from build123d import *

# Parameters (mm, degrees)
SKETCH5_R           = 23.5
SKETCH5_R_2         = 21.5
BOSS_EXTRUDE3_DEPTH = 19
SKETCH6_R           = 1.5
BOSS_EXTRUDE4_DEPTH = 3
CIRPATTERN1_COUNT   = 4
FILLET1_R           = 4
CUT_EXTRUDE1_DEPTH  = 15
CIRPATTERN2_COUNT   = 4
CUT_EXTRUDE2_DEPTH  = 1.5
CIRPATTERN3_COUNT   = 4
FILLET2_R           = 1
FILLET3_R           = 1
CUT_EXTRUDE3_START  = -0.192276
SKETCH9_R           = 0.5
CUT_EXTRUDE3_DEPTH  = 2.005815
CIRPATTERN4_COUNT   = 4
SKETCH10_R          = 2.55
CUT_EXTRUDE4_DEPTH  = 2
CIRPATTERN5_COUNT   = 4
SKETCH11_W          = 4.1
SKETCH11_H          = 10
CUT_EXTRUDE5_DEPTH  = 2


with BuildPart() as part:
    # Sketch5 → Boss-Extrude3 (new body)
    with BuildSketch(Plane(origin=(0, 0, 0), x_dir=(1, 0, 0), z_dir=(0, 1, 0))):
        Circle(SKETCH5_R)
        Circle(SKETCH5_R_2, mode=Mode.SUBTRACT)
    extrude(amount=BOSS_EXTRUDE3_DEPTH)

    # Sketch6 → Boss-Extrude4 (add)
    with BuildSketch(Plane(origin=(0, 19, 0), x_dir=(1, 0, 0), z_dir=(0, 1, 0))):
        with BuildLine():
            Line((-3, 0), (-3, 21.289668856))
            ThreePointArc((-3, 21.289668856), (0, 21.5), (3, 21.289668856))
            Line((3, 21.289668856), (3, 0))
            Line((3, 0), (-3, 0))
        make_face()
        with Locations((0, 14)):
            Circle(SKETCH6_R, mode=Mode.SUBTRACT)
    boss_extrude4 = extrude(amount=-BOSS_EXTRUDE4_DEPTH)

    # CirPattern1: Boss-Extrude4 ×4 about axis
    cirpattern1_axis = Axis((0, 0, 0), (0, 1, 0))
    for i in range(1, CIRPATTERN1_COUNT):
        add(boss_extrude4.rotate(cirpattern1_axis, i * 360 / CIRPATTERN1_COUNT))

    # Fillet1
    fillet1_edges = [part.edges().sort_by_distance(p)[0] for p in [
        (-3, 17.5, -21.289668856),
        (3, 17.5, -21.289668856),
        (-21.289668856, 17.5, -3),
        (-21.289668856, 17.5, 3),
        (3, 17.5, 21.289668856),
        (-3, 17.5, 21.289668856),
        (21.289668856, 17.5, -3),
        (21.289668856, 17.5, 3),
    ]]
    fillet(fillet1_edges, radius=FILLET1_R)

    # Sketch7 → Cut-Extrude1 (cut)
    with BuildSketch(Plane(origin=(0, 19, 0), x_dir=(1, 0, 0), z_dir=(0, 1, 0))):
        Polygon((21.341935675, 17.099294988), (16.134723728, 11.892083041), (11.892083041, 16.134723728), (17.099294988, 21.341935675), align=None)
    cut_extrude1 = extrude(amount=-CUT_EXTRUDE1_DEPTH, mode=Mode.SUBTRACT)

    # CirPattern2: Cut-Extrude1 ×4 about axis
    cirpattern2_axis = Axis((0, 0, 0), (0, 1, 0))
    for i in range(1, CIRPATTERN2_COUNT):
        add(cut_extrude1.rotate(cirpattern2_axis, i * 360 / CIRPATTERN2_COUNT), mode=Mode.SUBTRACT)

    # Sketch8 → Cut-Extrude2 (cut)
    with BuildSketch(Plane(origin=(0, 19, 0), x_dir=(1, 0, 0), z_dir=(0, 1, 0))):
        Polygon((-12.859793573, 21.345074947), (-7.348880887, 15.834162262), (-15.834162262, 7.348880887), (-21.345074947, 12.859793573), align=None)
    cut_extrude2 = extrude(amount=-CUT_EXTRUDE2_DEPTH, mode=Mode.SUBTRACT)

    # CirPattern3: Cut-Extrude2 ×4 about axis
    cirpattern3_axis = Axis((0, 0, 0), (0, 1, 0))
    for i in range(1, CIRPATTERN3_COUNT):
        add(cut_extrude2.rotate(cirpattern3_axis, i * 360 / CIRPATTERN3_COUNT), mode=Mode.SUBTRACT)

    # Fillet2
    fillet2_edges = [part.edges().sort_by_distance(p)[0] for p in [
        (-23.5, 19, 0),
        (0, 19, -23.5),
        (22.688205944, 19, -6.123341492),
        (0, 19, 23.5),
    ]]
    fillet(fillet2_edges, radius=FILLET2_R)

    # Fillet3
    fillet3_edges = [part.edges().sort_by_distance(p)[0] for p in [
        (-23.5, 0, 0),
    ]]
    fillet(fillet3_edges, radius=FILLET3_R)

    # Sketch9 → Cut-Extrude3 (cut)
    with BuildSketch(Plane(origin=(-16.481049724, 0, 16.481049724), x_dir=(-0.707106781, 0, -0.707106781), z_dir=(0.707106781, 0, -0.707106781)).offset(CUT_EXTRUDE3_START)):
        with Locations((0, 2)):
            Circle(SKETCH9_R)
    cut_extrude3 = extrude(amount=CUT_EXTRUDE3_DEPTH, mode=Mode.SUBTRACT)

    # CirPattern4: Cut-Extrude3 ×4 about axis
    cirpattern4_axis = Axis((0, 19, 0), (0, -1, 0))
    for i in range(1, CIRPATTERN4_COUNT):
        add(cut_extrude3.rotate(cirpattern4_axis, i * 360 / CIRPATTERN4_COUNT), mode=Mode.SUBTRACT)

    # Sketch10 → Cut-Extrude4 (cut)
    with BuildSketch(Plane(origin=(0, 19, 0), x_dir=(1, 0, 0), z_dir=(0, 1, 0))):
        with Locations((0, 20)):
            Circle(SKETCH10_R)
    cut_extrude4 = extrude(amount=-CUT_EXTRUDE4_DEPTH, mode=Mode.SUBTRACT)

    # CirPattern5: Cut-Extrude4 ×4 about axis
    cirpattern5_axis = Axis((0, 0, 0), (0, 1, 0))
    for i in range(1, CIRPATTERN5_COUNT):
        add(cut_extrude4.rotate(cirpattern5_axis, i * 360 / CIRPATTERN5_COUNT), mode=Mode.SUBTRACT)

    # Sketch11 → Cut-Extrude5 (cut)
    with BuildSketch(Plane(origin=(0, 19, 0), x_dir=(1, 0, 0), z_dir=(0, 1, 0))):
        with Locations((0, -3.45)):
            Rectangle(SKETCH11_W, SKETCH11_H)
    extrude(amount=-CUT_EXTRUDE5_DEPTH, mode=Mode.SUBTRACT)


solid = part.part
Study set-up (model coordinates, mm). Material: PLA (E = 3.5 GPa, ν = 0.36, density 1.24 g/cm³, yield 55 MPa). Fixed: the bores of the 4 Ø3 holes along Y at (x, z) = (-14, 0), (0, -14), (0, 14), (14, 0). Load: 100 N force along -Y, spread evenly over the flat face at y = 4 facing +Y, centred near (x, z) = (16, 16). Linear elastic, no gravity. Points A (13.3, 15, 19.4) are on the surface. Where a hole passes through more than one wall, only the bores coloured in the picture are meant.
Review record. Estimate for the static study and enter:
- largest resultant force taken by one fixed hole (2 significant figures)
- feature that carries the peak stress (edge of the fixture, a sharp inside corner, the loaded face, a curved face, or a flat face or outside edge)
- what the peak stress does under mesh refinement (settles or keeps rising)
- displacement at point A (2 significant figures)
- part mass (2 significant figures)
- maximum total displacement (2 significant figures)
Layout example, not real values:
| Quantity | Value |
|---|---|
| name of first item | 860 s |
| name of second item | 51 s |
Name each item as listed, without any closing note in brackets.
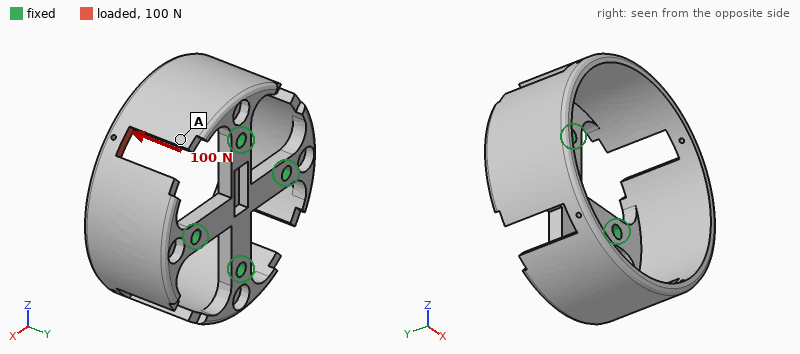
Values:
| Quantity | Value |
|---|---|
| largest resultant force taken by one fixed hole | 66 N |
| feature that carries the peak stress | a sharp inside corner |
| what the peak stress does under mesh refinement | keeps rising |
| displacement at point A | 0.50 mm |
| part mass | 7.2 g |
| maximum total displacement | 0.80 mm |
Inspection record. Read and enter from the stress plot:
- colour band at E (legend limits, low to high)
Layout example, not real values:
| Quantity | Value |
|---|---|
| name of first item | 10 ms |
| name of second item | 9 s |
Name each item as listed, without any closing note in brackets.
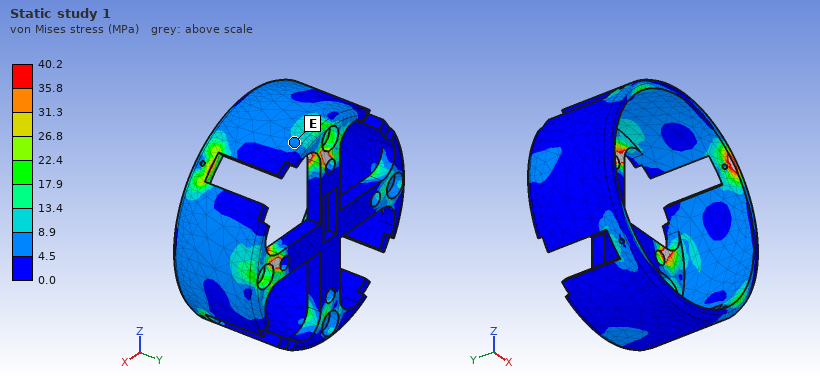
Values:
| Quantity | Value |
|---|---|
| colour band at E | 4.5 to 8.9 MPa |
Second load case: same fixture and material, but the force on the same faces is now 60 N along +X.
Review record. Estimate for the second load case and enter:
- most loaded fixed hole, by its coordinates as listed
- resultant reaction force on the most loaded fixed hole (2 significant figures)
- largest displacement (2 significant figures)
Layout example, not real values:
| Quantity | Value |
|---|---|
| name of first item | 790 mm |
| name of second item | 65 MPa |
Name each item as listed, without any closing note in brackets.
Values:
| Quantity | Value |
|---|---|
| most loaded fixed hole, by its coordinates as listed | (0, 14) |
| resultant reaction force on the most loaded fixed hole | 44 N |
| largest displacement | 0.71 mm |
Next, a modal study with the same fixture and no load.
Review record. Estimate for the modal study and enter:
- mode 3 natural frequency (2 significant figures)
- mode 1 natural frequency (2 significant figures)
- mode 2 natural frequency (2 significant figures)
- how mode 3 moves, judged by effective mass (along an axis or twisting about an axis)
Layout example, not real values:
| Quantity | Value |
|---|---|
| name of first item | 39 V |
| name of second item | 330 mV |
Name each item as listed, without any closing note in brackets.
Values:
| Quantity | Value |
|---|---|
| mode 3 natural frequency | 1800 Hz |
| mode 1 natural frequency | 1200 Hz |
| mode 2 natural frequency | 1600 Hz |
| how mode 3 moves, judged by effective mass | along X |
